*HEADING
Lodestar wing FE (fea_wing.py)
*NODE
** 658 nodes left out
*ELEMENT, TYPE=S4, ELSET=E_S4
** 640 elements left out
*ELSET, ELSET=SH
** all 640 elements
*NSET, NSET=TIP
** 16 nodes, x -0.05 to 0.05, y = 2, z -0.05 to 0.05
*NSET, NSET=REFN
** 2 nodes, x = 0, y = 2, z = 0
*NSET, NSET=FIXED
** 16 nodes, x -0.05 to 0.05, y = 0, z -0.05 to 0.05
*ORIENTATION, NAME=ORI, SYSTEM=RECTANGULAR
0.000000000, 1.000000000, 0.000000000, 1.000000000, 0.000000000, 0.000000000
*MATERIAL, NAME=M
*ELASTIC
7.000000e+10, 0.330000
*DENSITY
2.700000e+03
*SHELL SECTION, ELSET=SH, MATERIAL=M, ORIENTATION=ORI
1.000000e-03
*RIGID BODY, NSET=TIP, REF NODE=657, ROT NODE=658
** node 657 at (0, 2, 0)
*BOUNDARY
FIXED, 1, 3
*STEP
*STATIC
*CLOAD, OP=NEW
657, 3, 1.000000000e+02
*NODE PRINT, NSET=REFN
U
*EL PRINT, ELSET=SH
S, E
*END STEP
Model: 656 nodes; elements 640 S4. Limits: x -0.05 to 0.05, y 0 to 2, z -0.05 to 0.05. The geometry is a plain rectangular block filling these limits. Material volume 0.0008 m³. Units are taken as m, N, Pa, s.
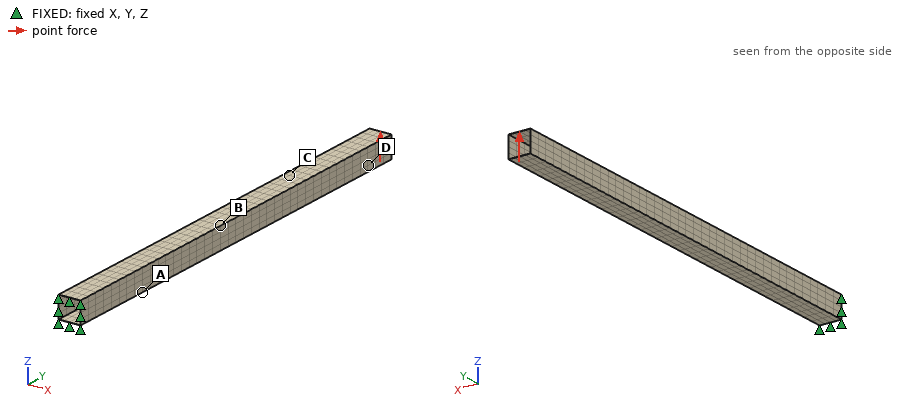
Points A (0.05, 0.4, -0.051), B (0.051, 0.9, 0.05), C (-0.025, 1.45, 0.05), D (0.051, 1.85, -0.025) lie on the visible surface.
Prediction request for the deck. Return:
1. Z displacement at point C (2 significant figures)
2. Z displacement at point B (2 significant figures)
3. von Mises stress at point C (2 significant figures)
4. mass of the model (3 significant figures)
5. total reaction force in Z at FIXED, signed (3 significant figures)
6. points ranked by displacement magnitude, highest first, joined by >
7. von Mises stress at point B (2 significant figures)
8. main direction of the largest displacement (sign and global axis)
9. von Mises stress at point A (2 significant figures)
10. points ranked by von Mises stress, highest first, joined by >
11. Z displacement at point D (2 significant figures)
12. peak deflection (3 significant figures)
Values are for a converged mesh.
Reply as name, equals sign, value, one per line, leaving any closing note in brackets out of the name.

Z displacement at point C = 0.0034 m
Z displacement at point B = 0.0015 m
von Mises stress at point C = 4.1e+06 Pa
mass of the model = 2.16 kg
total reaction force in Z at FIXED, signed = -100 N
points ranked by displacement magnitude, highest first, joined by > = D > C > B > A
von Mises stress at point B = 8.3e+06 Pa
main direction of the largest displacement = +Z
von Mises stress at point A = 1.2e+07 Pa
points ranked by von Mises stress, highest first, joined by > = A > B > C > D
Z displacement at point D = 0.0051 m
peak deflection = 0.00575 m
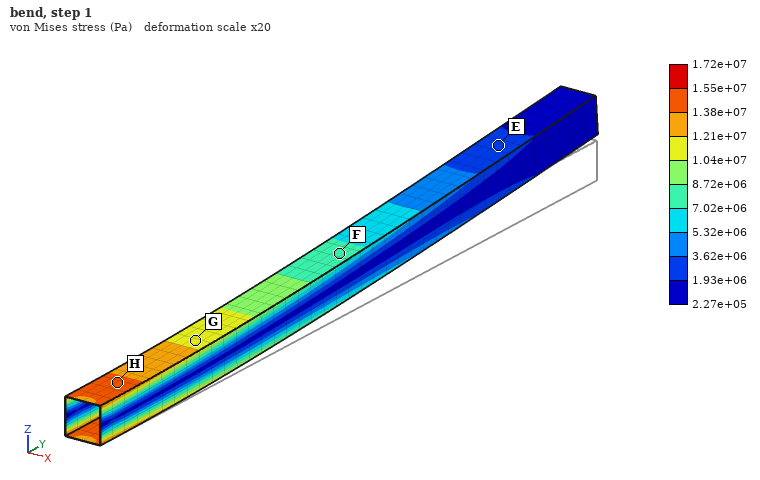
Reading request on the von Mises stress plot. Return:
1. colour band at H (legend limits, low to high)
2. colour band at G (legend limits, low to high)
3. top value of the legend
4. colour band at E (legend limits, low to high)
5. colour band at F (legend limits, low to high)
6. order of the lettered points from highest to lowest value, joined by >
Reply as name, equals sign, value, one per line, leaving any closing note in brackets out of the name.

colour band at H = 1.38e+07 to 1.55e+07 Pa
colour band at G = 1.04e+07 to 1.21e+07 Pa
top value of the legend = 1.72e+07 Pa
colour band at E = 1.93e+06 to 3.62e+06 Pa
colour band at F = 7.02e+06 to 8.72e+06 Pa
order of the lettered points from highest to lowest value, joined by > = H > G > F > E
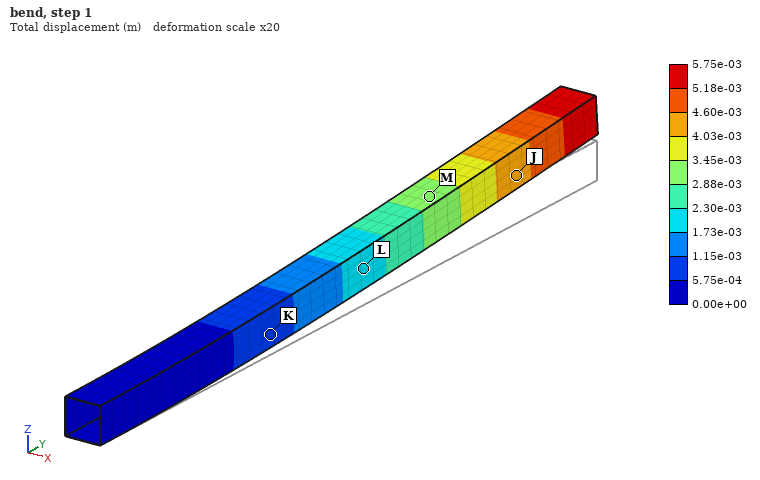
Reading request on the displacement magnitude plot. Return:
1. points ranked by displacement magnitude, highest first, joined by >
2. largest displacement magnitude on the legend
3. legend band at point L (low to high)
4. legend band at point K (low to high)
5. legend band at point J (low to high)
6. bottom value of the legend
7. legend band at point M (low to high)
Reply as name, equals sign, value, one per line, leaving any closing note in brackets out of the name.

points ranked by displacement magnitude, highest first, joined by > = J > M > L > K
largest displacement magnitude on the legend = 5.75e-03 m
legend band at point L = 1.73e-03 to 2.30e-03 m
legend band at point K = 5.75e-04 to 1.15e-03 m
legend band at point J = 4.03e-03 to 4.60e-03 m
bottom value of the legend = 0.00e+00 m
legend band at point M = 2.88e-03 to 3.45e-03 m
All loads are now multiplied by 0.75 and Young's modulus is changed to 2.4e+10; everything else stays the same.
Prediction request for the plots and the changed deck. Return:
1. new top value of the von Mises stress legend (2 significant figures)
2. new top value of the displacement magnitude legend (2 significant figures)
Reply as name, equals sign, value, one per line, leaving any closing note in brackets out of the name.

new top value of the von Mises stress legend = 1.3e+07 Pa
new top value of the displacement magnitude legend = 0.013 m
